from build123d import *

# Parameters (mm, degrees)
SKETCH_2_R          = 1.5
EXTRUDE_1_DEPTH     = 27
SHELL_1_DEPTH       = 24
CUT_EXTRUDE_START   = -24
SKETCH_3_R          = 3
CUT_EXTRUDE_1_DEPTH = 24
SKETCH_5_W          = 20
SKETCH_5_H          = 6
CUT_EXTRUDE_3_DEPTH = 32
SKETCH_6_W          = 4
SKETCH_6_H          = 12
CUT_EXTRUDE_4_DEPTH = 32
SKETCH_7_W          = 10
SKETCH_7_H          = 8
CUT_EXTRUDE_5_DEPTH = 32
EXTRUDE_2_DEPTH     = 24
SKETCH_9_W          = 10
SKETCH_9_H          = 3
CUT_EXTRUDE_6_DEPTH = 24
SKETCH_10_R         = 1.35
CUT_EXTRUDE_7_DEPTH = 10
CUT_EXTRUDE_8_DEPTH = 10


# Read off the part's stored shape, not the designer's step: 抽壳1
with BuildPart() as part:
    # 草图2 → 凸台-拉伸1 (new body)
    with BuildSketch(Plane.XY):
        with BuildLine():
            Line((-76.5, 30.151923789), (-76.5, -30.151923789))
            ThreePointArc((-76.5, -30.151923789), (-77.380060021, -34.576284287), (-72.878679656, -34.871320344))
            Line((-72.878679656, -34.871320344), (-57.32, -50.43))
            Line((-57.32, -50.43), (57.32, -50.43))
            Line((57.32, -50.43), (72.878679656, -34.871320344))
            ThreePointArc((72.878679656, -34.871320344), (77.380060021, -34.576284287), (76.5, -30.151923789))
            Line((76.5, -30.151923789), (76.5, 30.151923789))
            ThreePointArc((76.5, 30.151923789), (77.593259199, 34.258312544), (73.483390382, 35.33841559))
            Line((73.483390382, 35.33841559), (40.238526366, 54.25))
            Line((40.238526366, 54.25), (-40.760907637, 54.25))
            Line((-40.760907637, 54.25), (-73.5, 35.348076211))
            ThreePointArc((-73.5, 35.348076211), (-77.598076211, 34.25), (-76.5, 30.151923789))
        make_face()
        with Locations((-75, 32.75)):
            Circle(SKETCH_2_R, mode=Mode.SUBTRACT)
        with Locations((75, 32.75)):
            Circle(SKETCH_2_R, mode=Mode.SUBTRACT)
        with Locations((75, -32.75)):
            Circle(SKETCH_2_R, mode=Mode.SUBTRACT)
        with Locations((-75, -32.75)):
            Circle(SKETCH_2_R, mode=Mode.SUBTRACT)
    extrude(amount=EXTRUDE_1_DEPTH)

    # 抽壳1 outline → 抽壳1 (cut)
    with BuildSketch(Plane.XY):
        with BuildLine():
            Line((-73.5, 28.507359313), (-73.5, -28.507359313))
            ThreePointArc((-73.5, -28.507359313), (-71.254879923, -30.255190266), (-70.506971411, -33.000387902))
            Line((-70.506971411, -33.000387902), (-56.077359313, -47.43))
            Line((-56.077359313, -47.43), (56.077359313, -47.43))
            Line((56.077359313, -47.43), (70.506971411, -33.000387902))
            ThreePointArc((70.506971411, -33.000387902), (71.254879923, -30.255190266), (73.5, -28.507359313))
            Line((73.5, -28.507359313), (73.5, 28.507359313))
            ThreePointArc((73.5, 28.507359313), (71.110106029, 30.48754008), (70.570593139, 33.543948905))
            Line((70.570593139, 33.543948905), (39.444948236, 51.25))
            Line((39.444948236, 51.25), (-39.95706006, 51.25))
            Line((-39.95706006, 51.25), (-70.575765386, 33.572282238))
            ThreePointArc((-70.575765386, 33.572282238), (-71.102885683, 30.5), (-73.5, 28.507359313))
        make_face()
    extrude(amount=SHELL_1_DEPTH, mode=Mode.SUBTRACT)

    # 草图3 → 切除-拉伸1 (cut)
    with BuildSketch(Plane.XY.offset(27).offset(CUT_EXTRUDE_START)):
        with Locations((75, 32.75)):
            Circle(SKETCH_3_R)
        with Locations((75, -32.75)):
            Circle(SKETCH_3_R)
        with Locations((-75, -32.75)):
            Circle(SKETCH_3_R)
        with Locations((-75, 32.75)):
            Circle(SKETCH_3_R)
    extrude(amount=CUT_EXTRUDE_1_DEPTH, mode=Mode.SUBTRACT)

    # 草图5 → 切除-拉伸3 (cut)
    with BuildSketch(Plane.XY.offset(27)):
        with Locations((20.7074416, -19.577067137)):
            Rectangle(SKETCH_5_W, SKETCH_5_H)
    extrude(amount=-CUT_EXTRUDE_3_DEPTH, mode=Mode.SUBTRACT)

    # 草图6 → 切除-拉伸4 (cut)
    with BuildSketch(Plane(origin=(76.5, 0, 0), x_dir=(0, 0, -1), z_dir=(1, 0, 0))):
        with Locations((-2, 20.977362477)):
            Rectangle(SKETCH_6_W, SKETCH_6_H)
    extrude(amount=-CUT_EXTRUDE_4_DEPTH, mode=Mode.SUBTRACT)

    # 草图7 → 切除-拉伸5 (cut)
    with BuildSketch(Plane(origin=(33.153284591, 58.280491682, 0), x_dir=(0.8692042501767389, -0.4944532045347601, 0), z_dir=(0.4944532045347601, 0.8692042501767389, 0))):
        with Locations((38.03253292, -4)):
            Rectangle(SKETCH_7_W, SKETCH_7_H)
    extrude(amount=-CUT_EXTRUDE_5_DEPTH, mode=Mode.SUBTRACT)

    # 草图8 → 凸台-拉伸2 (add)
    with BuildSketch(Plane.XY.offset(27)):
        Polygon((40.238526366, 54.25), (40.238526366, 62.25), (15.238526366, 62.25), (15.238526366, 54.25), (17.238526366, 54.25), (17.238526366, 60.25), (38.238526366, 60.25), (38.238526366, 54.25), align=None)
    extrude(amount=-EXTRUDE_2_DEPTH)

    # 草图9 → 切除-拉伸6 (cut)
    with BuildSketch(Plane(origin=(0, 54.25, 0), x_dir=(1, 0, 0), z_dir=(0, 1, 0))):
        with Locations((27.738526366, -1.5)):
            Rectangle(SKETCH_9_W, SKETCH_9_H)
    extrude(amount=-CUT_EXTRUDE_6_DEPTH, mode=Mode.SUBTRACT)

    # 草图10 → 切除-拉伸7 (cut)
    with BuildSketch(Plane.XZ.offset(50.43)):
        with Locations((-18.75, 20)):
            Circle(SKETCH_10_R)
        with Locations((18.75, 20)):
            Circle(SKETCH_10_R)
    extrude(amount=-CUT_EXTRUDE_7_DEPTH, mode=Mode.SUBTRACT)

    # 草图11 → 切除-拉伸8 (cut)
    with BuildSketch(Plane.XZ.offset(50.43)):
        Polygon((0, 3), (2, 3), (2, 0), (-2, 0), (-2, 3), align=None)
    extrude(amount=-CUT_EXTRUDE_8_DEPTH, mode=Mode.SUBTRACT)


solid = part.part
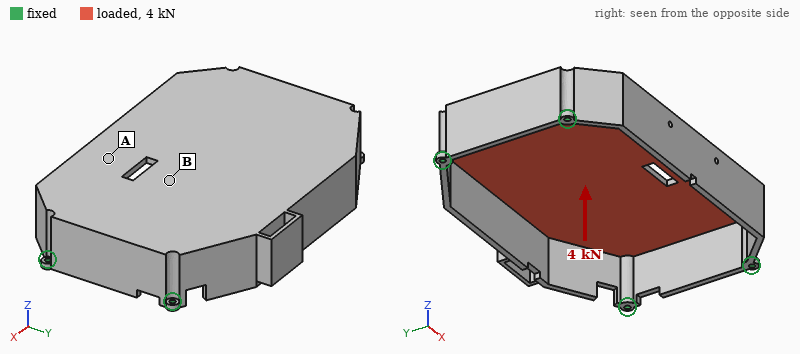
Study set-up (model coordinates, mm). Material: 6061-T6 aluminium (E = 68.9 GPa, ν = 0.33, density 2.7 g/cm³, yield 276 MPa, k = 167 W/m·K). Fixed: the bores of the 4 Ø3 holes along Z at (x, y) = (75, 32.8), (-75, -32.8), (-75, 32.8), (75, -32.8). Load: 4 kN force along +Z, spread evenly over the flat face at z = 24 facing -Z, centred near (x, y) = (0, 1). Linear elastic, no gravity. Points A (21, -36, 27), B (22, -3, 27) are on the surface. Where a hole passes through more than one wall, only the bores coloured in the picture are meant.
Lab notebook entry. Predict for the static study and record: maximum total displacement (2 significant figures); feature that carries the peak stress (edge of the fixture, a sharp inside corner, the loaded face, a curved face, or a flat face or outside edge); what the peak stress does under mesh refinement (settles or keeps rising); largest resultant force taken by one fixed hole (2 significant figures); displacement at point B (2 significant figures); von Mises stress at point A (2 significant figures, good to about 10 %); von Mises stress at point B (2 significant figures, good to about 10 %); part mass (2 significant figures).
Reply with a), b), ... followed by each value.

a) 0.75 mm
b) edge of the fixture
c) keeps rising
d) 1.2 kN
e) 0.66 mm
f) 37 MPa
g) 72 MPa
h) 210 g
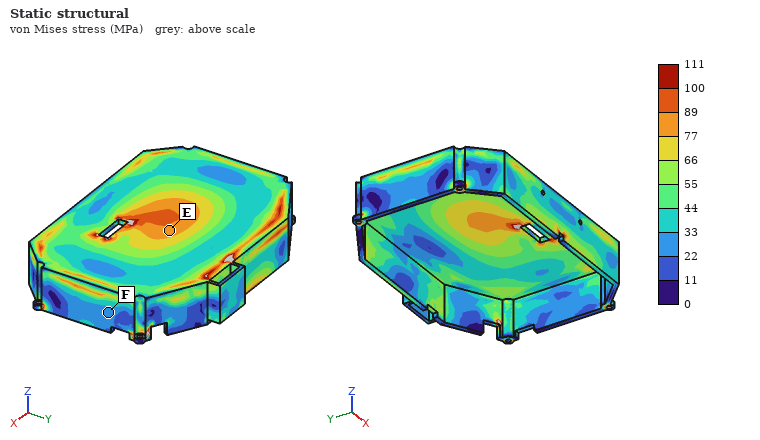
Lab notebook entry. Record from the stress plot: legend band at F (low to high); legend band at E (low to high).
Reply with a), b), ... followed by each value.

a) 22 to 33 MPa
b) 77 to 89 MPa
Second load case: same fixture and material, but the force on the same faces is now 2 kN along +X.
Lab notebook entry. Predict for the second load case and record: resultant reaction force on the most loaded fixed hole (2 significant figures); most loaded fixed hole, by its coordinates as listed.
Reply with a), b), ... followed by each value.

a) 680 N
b) (-75, 32.8)
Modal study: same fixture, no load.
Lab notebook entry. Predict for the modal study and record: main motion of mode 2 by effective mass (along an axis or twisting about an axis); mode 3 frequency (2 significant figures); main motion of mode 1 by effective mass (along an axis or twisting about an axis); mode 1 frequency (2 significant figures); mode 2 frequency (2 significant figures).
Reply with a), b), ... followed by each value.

a) along X
b) 2300 Hz
c) along Z
d) 1400 Hz
e) 1700 Hz
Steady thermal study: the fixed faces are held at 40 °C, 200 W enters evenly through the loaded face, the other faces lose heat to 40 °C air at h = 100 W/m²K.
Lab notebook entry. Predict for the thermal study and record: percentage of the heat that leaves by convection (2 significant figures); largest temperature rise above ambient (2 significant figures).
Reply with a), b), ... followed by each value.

a) 74 %
b) 57 K
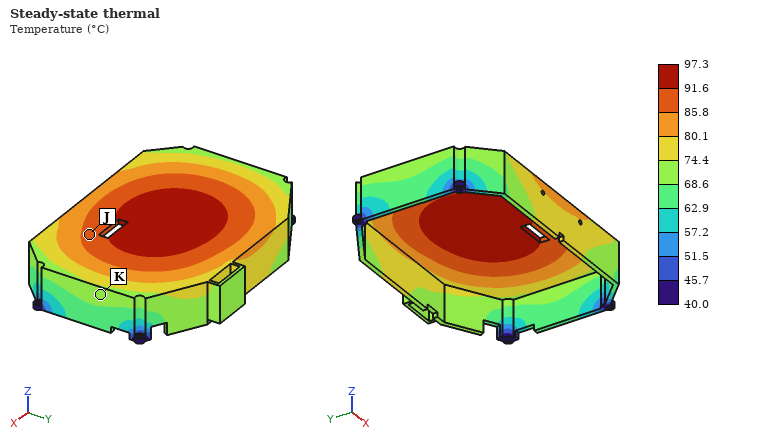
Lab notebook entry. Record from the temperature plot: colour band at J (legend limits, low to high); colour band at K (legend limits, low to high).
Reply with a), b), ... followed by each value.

a) 85.8 to 91.6 °C
b) 68.6 to 74.4 °C
